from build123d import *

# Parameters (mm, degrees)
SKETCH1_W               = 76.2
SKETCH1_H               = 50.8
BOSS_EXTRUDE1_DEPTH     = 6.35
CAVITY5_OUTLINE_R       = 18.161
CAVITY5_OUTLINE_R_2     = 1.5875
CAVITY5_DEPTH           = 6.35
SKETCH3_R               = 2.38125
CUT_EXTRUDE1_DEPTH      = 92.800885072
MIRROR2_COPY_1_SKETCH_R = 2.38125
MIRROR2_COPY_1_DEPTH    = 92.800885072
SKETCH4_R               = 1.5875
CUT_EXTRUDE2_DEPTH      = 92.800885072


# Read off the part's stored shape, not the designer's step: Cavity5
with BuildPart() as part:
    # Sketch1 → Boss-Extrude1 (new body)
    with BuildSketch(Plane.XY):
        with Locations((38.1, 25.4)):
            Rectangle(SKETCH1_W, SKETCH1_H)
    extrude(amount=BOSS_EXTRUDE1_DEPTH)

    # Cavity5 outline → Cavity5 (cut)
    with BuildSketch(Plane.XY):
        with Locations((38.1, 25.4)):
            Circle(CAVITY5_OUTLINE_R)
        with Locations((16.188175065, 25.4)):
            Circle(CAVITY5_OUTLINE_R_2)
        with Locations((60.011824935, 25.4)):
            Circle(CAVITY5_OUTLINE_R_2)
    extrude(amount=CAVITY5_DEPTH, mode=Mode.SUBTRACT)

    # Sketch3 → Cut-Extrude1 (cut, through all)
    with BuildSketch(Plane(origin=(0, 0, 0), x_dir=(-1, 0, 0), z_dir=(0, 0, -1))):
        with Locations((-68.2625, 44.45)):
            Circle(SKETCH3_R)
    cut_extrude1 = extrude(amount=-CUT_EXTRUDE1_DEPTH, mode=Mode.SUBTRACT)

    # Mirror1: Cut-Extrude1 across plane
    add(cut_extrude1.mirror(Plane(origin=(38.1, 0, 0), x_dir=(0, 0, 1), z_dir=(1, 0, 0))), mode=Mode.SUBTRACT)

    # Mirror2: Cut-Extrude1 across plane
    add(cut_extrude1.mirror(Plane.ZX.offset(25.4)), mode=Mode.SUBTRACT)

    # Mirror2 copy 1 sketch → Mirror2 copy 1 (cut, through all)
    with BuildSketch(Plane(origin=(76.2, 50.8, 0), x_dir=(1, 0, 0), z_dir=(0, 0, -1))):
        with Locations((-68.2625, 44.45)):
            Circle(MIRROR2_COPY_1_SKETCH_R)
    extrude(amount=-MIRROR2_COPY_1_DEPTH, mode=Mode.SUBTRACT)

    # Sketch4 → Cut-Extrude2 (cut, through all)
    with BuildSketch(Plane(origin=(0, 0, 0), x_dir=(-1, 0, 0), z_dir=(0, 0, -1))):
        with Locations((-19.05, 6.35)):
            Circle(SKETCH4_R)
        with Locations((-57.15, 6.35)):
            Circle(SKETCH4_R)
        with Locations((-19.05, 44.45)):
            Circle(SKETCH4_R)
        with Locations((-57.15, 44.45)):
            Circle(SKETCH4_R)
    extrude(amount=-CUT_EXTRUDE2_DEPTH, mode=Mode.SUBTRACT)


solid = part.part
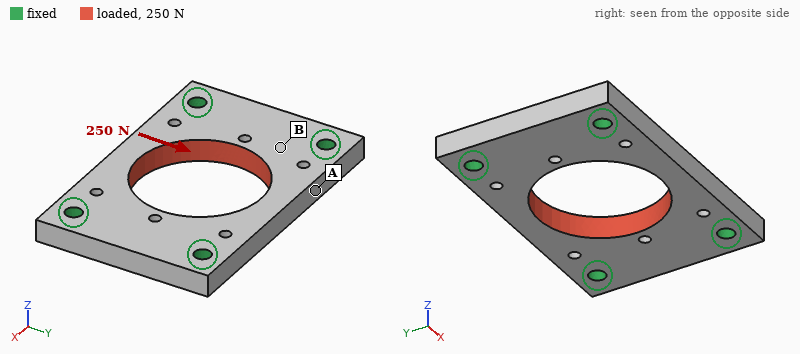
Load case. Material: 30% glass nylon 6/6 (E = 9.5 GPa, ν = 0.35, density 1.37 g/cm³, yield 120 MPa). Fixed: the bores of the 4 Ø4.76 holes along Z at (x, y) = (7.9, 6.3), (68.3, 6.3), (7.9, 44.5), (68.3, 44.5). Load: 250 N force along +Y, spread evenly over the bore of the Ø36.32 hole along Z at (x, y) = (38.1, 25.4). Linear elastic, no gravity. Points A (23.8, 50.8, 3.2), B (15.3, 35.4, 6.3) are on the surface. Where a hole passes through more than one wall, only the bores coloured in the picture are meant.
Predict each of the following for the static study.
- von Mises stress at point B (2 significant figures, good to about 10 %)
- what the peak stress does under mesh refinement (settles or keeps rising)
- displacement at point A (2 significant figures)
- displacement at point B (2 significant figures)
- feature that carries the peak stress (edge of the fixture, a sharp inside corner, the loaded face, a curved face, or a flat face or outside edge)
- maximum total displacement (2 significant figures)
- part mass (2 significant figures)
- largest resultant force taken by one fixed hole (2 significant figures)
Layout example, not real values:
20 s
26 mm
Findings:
0.97 MPa
keeps rising
3.5 µm
1.4 µm
edge of the fixture
6.5 µm
24 g
67 N
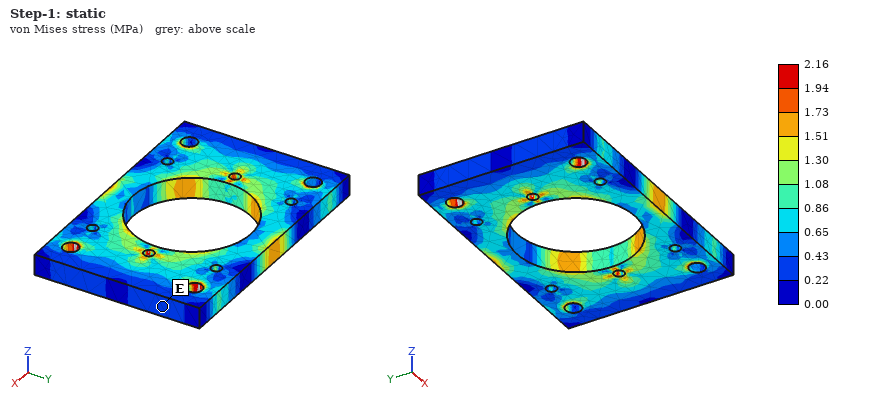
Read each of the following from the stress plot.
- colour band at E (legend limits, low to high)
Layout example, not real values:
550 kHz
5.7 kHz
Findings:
0.22 to 0.43 MPa
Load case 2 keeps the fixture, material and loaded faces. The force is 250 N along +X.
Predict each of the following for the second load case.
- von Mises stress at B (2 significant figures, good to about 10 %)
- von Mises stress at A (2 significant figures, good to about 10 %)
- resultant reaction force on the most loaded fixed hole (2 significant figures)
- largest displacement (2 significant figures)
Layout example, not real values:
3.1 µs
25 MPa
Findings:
0.42 MPa
0.51 MPa
64 N
1.7 µm
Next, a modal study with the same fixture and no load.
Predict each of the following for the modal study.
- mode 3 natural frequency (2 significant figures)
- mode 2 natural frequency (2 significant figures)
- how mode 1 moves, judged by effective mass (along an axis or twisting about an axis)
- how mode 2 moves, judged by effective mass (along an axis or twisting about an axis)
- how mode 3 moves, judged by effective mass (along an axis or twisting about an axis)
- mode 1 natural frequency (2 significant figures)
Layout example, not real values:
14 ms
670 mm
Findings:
8900 Hz
5500 Hz
along Z
twisting about X
twisting about Y
5200 Hz
